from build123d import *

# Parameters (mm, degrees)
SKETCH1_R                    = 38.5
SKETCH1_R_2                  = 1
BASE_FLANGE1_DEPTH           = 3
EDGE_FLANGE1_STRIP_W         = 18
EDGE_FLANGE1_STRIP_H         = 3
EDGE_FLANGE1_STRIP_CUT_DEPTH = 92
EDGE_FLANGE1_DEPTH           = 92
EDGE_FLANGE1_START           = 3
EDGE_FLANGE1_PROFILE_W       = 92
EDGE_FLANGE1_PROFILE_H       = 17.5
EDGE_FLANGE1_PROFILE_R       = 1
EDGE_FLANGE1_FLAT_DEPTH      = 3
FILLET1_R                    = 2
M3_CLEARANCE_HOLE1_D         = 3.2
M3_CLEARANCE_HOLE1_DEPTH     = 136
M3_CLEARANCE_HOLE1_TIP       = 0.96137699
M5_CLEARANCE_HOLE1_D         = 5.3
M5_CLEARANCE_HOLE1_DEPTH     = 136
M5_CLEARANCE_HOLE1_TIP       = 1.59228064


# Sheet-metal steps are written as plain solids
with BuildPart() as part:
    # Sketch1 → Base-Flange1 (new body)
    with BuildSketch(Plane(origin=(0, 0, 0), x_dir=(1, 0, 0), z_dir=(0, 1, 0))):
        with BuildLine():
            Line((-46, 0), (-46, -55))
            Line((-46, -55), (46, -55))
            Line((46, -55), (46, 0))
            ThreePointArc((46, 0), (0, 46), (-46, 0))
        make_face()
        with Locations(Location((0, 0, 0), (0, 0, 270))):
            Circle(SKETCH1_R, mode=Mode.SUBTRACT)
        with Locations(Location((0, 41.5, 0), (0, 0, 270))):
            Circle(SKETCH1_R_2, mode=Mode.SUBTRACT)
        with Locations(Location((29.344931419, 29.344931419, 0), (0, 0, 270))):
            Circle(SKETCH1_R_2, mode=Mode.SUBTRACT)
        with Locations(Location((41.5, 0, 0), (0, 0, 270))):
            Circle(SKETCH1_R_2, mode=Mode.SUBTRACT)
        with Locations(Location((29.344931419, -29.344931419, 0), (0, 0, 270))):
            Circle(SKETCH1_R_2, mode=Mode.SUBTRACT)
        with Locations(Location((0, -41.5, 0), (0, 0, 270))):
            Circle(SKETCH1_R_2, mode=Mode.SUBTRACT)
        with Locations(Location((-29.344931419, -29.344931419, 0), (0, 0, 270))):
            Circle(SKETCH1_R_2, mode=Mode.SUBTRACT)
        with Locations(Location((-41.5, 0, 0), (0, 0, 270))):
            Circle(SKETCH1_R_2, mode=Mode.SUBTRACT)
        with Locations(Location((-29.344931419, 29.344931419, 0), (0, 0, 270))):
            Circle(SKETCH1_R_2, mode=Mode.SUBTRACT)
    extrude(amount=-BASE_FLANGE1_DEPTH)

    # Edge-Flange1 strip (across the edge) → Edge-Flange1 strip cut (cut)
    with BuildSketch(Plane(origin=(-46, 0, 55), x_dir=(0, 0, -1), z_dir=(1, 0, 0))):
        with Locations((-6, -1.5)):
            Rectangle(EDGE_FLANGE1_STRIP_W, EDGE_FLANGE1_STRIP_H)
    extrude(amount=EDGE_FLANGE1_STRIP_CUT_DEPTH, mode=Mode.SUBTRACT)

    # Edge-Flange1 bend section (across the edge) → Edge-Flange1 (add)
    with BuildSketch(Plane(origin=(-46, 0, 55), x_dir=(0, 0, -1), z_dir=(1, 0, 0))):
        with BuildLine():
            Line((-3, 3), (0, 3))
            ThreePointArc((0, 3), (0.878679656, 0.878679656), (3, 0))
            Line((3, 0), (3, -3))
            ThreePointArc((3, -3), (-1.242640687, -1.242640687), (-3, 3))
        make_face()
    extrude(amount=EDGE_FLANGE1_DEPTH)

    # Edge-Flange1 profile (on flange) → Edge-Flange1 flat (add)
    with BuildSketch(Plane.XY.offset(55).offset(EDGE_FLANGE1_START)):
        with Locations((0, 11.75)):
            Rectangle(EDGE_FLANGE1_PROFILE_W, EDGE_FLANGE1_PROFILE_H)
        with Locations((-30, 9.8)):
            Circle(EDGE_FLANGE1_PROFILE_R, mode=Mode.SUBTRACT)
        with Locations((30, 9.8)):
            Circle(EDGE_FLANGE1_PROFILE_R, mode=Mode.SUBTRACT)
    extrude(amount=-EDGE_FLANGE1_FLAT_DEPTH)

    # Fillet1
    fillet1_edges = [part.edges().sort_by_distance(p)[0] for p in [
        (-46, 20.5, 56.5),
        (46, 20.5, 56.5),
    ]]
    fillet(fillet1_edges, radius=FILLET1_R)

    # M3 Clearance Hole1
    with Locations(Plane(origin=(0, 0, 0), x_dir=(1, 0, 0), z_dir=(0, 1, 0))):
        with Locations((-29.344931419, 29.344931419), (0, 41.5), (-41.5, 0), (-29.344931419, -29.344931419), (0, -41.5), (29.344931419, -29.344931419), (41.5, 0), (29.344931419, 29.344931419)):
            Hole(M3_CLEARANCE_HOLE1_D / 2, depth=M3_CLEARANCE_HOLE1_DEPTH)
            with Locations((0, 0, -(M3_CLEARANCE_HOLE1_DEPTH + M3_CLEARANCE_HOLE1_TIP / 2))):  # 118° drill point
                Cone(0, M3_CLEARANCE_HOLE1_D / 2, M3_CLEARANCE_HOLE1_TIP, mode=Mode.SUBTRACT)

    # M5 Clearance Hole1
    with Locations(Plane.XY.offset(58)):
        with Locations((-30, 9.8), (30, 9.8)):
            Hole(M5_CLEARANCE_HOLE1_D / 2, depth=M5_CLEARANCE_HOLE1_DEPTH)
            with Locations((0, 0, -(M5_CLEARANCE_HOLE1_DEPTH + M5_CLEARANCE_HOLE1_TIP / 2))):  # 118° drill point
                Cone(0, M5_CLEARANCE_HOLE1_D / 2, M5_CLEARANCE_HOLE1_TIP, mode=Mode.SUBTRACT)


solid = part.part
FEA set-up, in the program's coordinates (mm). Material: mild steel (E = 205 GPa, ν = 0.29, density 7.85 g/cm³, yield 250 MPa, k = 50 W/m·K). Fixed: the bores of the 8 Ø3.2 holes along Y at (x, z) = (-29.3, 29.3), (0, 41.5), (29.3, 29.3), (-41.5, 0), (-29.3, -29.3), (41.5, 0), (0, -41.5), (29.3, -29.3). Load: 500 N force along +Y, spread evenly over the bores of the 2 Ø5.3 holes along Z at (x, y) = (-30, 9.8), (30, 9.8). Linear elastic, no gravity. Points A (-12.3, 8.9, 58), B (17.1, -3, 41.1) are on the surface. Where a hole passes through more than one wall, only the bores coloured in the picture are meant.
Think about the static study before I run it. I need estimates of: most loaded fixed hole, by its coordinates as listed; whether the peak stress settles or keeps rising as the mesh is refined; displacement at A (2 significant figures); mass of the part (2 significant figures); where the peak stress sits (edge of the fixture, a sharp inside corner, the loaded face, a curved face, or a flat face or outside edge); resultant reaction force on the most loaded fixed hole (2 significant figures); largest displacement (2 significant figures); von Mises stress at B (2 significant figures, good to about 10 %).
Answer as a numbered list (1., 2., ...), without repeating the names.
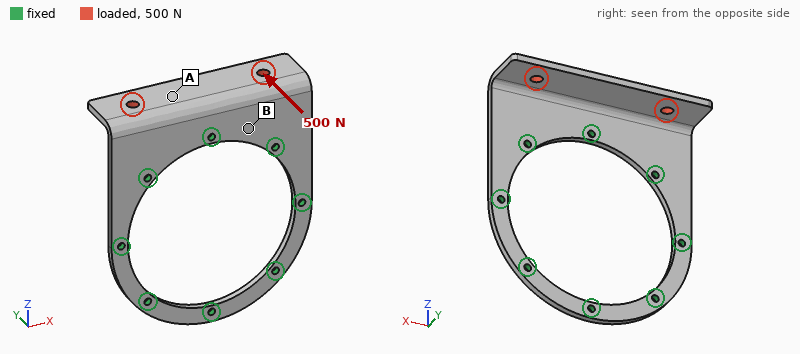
1. (0, 41.5)
2. keeps rising
3. 52 µm
4. 130 g
5. edge of the fixture
6. 520 N
7. 76 µm
8. 22 MPa
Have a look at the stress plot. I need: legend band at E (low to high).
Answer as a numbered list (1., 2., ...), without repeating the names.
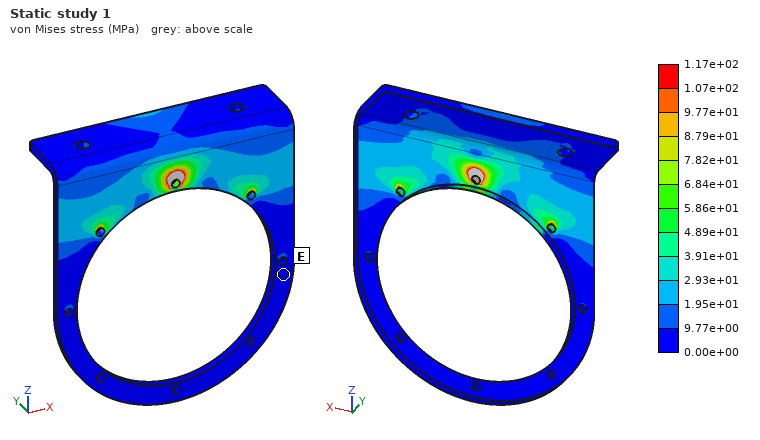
1. 0.00e+00 to 9.77e+00 MPa
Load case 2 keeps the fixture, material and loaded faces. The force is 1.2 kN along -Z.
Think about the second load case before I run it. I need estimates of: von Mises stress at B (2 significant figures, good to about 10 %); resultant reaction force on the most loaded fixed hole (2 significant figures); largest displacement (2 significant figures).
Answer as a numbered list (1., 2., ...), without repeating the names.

1. 51 MPa
2. 510 N
3. 0.18 mm
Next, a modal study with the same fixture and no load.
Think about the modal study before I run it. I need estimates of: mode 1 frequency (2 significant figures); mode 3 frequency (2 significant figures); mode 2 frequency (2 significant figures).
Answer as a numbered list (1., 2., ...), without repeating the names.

1. 1800 Hz
2. 4600 Hz
3. 1800 Hz
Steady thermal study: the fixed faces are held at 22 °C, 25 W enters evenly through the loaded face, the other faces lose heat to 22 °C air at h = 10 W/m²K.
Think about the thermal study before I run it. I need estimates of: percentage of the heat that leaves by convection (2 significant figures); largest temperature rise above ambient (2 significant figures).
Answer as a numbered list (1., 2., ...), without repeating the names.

1. 15 %
2. 85 K
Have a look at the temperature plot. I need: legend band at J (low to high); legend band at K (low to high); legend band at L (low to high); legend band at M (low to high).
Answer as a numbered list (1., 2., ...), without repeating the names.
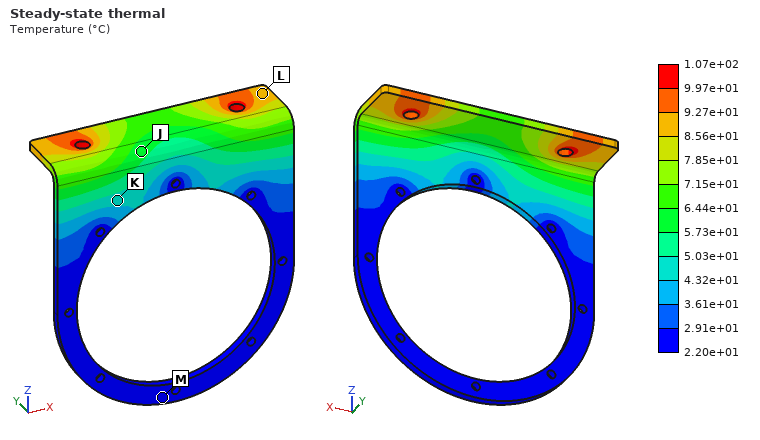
1. 5.73e+01 to 6.44e+01 °C
2. 4.32e+01 to 5.03e+01 °C
3. 8.56e+01 to 9.27e+01 °C
4. 2.20e+01 to 2.91e+01 °C
